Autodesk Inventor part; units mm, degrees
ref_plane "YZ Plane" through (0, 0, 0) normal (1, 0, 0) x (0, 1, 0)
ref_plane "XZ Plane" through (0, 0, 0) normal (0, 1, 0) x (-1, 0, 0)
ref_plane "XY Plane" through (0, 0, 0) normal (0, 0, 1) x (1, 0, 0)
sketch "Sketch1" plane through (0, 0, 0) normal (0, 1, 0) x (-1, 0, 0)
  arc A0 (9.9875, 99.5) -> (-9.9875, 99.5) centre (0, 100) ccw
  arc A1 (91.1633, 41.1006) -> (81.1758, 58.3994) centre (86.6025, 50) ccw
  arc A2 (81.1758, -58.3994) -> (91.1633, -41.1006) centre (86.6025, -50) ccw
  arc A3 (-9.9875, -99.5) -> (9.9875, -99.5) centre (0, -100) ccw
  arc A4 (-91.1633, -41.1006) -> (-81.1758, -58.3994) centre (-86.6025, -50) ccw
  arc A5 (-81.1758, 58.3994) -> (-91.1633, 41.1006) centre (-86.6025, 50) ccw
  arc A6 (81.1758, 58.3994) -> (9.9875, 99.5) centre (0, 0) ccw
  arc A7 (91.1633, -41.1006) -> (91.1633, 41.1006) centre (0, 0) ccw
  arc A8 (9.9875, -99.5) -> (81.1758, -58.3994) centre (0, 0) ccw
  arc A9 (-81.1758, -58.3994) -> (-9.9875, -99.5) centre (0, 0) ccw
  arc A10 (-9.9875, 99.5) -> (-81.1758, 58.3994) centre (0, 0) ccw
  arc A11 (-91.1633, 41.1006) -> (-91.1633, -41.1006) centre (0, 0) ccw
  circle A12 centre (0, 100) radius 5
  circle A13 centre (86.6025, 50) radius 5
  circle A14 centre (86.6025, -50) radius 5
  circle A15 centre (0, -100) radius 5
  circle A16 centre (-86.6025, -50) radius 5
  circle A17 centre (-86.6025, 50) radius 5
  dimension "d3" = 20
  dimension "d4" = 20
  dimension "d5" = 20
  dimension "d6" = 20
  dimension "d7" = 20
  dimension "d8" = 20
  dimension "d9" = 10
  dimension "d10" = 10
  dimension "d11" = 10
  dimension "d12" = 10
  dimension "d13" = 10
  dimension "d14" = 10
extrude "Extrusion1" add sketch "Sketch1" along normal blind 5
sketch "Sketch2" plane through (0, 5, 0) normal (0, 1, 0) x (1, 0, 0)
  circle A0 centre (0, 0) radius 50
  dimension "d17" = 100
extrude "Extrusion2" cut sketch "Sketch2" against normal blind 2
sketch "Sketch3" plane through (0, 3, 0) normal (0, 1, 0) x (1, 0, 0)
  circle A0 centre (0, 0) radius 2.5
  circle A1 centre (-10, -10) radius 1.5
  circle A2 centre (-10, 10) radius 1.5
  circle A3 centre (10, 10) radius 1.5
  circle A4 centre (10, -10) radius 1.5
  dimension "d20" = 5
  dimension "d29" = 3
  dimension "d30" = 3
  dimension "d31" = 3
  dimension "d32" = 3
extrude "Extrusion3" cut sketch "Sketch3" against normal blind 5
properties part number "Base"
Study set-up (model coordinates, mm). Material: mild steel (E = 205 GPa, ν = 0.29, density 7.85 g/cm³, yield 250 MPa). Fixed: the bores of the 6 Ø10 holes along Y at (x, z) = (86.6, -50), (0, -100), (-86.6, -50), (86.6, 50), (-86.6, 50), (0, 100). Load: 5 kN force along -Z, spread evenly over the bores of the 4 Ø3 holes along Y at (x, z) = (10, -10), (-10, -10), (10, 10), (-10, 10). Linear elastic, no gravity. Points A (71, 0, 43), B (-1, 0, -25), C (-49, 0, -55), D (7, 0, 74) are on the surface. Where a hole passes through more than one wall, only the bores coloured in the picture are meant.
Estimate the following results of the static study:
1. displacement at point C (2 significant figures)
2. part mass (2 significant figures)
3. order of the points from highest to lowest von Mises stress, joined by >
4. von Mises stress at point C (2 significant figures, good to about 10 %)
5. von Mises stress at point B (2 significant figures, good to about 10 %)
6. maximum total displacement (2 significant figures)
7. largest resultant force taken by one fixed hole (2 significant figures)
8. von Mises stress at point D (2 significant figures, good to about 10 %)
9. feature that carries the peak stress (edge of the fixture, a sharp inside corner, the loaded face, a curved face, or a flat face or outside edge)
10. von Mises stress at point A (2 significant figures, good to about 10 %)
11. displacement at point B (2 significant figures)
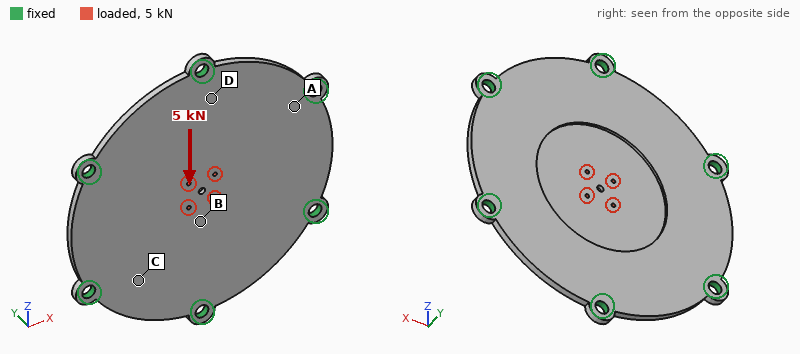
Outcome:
1.4 µm
1.1 kg
B > D > A > C
2.9 MPa
12 MPa
5.6 µm
1.3 kN
9.1 MPa
the loaded face
5.6 MPa
4.7 µm
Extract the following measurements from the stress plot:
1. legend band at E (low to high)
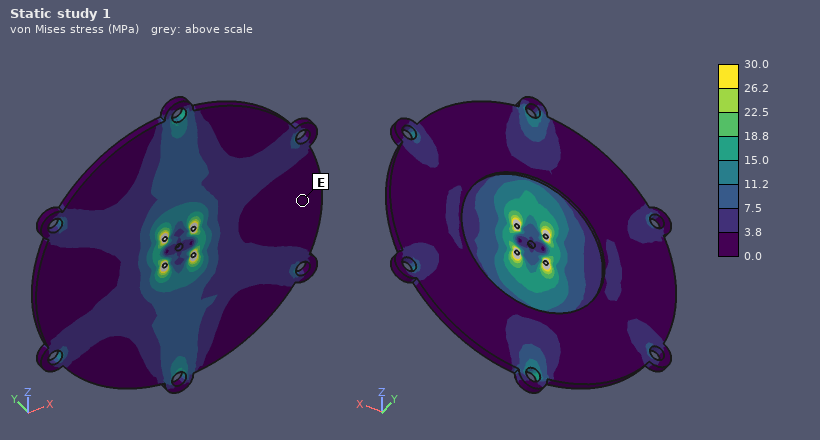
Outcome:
0.0 to 3.8 MPa
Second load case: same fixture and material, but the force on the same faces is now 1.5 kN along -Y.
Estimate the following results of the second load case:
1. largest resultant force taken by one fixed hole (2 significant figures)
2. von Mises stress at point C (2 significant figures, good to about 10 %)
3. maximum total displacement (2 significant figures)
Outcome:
950 N
23 MPa
0.30 mm
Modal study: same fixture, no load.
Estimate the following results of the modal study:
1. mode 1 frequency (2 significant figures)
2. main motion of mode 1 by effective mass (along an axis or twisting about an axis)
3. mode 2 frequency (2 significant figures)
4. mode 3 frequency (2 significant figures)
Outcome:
1000 Hz
along Y
1900 Hz
1900 Hz
